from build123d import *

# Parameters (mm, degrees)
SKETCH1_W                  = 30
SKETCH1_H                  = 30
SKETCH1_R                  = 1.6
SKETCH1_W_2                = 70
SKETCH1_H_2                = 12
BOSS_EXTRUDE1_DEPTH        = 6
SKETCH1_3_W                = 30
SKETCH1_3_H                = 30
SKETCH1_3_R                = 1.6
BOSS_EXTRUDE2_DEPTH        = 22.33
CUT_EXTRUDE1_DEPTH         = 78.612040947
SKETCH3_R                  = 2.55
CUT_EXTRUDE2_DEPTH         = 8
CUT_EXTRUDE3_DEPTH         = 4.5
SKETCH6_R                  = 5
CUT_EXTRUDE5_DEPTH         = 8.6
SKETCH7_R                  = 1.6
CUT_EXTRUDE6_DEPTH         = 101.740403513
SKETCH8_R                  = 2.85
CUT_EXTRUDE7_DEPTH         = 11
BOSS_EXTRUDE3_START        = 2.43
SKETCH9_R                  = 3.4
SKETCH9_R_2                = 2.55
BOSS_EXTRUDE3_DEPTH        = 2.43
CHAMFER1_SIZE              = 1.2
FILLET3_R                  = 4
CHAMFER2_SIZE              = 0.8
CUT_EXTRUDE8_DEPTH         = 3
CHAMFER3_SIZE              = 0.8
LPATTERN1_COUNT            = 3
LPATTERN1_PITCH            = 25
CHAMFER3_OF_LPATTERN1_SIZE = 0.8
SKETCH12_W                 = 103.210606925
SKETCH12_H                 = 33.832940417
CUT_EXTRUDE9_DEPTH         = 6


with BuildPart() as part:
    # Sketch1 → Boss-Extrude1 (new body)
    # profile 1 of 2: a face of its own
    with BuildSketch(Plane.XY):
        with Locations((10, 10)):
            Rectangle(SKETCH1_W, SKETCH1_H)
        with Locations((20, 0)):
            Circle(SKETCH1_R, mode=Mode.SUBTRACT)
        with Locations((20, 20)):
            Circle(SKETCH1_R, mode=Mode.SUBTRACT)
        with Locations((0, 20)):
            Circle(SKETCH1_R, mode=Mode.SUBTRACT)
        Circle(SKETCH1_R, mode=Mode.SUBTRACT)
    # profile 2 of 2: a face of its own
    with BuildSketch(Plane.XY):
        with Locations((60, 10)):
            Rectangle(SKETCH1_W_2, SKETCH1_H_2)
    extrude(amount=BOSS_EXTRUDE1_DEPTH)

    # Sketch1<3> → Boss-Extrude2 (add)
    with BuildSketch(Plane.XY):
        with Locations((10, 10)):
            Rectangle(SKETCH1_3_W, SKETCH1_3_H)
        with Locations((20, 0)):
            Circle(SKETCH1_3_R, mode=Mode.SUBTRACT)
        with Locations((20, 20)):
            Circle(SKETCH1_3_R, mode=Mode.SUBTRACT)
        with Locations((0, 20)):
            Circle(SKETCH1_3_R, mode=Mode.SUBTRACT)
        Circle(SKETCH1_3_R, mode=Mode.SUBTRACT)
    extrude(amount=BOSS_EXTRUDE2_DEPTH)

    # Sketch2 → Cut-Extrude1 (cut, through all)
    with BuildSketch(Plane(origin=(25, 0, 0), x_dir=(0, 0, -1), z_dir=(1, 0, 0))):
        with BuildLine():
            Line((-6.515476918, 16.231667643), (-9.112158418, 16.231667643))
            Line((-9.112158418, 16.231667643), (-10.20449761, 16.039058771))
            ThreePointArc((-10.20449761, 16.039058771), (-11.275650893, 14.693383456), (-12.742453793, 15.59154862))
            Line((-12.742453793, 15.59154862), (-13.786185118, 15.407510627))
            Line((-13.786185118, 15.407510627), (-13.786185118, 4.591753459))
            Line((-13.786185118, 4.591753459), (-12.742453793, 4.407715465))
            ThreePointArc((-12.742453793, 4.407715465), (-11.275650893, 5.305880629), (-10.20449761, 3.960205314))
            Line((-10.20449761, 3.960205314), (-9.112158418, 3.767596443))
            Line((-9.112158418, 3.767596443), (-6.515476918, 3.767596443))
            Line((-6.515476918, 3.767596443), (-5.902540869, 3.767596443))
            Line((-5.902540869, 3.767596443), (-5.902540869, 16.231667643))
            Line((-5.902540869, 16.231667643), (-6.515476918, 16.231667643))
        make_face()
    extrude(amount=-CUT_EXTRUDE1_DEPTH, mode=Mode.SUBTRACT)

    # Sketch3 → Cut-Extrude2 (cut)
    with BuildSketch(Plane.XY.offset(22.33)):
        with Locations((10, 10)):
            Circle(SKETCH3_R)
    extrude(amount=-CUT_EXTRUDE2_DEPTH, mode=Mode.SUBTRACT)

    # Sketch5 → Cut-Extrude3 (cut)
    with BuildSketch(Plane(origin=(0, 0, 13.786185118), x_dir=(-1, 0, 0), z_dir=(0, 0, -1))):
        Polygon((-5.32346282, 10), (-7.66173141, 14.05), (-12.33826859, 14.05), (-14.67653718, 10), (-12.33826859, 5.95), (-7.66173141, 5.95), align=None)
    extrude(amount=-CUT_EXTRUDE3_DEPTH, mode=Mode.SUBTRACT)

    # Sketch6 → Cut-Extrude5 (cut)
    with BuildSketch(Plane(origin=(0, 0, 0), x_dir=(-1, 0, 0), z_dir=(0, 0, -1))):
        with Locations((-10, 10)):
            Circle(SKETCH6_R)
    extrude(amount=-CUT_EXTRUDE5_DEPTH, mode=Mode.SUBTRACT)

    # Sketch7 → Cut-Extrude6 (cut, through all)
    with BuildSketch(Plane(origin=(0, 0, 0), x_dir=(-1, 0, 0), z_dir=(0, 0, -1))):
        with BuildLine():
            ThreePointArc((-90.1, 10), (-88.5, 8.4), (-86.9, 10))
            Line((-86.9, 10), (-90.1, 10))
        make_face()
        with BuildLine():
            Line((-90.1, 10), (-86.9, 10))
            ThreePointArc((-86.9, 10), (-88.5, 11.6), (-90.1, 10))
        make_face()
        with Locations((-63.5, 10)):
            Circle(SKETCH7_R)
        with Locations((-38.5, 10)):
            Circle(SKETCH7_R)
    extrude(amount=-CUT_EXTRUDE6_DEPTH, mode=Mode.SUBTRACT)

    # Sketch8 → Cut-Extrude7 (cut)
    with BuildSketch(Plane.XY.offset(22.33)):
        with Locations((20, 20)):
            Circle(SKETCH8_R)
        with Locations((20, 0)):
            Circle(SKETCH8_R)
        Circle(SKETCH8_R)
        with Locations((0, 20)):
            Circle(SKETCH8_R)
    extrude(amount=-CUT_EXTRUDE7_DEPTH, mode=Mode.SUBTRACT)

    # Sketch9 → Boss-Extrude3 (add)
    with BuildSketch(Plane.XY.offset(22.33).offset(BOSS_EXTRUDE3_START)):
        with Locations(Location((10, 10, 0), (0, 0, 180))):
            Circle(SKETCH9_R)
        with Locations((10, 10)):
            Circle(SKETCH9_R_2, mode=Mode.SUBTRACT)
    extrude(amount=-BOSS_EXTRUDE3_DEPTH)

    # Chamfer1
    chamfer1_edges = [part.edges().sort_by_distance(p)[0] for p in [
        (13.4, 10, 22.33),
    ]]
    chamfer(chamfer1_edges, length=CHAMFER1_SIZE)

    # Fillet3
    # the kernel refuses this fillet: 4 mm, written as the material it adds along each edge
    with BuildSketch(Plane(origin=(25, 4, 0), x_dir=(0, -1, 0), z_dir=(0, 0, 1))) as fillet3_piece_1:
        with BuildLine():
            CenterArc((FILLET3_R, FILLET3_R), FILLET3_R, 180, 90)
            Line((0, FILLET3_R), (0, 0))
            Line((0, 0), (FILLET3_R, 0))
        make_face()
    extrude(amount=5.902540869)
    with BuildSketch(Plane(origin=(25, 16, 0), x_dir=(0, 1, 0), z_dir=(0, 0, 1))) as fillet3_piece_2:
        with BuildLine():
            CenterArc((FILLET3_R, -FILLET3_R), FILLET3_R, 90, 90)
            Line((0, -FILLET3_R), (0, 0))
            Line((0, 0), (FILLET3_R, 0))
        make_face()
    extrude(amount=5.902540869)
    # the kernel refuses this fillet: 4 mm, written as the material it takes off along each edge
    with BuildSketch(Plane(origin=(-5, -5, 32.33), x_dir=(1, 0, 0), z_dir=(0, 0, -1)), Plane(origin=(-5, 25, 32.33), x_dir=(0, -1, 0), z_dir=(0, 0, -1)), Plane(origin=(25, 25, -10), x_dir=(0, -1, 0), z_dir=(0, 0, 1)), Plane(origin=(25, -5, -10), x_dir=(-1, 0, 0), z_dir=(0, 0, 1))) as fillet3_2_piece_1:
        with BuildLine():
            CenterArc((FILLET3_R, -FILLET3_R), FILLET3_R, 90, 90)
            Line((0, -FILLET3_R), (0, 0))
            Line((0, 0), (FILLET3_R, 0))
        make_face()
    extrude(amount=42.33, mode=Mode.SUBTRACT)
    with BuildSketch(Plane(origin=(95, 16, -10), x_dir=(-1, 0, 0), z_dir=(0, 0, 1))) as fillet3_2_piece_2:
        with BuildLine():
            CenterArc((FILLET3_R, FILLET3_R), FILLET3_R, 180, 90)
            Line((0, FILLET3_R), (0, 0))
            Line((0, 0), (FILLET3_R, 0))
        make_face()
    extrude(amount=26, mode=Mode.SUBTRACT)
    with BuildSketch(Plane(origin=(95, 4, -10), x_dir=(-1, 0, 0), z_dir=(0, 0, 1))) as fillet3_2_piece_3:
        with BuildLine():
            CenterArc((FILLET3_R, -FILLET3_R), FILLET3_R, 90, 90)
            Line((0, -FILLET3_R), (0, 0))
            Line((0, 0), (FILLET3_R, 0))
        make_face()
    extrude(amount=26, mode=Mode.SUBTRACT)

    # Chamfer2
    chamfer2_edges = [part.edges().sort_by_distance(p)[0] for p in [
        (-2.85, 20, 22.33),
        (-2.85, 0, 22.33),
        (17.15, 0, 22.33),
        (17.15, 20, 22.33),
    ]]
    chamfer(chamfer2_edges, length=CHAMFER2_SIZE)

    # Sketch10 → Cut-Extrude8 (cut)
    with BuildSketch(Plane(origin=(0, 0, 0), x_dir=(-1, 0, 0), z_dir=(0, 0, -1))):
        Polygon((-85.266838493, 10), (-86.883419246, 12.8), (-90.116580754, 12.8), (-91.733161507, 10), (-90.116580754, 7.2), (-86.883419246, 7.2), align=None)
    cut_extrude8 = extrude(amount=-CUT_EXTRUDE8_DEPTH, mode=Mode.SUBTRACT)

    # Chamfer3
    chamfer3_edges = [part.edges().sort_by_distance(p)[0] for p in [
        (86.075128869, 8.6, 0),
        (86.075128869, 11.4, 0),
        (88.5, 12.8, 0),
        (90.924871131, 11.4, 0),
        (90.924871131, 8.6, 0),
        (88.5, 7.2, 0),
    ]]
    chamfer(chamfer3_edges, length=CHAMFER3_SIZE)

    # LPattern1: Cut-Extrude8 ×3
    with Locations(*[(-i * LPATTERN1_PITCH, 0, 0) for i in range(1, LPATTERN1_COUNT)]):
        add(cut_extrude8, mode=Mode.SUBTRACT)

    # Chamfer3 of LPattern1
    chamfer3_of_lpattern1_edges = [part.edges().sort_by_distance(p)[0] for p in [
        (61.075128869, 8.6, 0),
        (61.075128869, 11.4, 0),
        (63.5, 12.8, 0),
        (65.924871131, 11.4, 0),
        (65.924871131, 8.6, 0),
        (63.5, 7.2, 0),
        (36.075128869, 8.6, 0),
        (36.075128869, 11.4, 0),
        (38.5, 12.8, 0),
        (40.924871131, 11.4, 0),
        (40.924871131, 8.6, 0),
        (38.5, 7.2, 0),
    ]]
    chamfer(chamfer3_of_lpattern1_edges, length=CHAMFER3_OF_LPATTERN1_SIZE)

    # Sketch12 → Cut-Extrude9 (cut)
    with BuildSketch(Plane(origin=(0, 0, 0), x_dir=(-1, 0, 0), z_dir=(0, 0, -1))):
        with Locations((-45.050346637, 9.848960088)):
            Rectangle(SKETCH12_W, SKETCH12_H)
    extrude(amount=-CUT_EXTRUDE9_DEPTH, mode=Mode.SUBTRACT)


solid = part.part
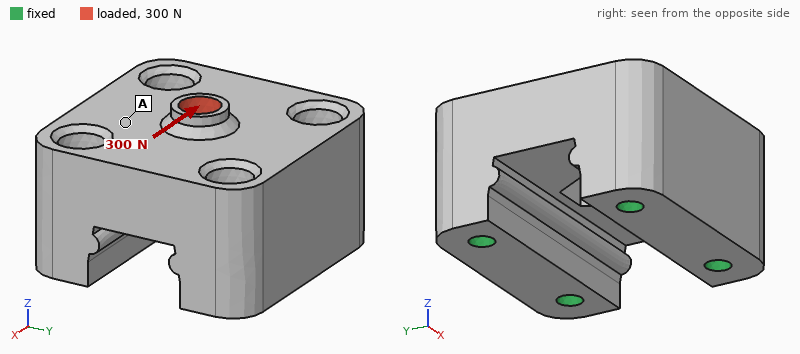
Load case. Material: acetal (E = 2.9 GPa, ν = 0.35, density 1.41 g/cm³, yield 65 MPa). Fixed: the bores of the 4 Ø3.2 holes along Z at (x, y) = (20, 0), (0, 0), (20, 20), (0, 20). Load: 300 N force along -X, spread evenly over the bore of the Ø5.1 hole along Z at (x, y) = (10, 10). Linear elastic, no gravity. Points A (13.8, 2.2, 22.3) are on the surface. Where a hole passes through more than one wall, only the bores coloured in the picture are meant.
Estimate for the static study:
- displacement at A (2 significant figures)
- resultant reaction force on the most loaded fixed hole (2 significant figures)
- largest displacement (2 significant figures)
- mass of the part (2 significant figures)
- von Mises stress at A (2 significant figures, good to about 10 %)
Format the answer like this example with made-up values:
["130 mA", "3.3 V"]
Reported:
["15 µm", "120 N", "43 µm", "14 g", "1.5 MPa"]
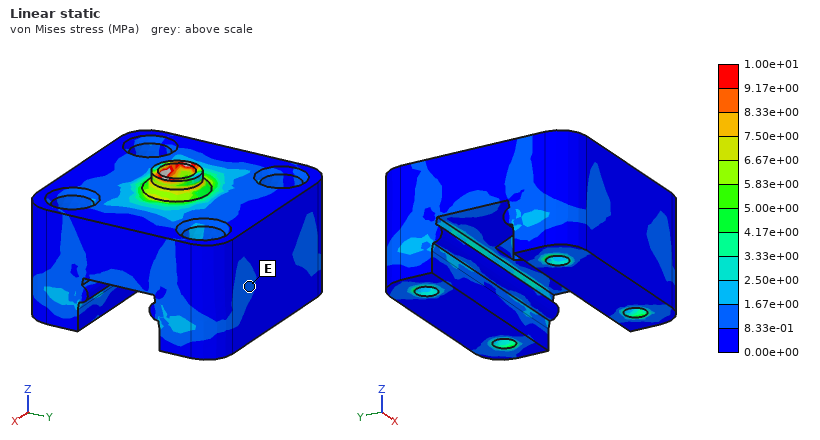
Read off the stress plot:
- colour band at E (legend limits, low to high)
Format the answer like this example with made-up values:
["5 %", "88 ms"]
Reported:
["8.33e-01 to 1.67e+00 MPa"]
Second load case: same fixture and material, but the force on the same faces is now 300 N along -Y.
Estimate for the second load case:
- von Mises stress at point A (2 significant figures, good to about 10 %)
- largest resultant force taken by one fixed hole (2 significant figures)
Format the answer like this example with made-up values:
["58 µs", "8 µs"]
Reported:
["1.8 MPa", "110 N"]
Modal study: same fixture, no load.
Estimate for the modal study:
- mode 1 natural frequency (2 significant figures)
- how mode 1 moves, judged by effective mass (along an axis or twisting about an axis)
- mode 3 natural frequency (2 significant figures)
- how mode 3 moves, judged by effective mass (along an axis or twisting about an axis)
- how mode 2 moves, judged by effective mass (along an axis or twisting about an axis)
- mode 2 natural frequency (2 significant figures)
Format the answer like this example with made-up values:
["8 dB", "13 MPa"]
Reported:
["7000 Hz", "along Y", "11 kHz", "twisting about Z", "along X", "8600 Hz"]
